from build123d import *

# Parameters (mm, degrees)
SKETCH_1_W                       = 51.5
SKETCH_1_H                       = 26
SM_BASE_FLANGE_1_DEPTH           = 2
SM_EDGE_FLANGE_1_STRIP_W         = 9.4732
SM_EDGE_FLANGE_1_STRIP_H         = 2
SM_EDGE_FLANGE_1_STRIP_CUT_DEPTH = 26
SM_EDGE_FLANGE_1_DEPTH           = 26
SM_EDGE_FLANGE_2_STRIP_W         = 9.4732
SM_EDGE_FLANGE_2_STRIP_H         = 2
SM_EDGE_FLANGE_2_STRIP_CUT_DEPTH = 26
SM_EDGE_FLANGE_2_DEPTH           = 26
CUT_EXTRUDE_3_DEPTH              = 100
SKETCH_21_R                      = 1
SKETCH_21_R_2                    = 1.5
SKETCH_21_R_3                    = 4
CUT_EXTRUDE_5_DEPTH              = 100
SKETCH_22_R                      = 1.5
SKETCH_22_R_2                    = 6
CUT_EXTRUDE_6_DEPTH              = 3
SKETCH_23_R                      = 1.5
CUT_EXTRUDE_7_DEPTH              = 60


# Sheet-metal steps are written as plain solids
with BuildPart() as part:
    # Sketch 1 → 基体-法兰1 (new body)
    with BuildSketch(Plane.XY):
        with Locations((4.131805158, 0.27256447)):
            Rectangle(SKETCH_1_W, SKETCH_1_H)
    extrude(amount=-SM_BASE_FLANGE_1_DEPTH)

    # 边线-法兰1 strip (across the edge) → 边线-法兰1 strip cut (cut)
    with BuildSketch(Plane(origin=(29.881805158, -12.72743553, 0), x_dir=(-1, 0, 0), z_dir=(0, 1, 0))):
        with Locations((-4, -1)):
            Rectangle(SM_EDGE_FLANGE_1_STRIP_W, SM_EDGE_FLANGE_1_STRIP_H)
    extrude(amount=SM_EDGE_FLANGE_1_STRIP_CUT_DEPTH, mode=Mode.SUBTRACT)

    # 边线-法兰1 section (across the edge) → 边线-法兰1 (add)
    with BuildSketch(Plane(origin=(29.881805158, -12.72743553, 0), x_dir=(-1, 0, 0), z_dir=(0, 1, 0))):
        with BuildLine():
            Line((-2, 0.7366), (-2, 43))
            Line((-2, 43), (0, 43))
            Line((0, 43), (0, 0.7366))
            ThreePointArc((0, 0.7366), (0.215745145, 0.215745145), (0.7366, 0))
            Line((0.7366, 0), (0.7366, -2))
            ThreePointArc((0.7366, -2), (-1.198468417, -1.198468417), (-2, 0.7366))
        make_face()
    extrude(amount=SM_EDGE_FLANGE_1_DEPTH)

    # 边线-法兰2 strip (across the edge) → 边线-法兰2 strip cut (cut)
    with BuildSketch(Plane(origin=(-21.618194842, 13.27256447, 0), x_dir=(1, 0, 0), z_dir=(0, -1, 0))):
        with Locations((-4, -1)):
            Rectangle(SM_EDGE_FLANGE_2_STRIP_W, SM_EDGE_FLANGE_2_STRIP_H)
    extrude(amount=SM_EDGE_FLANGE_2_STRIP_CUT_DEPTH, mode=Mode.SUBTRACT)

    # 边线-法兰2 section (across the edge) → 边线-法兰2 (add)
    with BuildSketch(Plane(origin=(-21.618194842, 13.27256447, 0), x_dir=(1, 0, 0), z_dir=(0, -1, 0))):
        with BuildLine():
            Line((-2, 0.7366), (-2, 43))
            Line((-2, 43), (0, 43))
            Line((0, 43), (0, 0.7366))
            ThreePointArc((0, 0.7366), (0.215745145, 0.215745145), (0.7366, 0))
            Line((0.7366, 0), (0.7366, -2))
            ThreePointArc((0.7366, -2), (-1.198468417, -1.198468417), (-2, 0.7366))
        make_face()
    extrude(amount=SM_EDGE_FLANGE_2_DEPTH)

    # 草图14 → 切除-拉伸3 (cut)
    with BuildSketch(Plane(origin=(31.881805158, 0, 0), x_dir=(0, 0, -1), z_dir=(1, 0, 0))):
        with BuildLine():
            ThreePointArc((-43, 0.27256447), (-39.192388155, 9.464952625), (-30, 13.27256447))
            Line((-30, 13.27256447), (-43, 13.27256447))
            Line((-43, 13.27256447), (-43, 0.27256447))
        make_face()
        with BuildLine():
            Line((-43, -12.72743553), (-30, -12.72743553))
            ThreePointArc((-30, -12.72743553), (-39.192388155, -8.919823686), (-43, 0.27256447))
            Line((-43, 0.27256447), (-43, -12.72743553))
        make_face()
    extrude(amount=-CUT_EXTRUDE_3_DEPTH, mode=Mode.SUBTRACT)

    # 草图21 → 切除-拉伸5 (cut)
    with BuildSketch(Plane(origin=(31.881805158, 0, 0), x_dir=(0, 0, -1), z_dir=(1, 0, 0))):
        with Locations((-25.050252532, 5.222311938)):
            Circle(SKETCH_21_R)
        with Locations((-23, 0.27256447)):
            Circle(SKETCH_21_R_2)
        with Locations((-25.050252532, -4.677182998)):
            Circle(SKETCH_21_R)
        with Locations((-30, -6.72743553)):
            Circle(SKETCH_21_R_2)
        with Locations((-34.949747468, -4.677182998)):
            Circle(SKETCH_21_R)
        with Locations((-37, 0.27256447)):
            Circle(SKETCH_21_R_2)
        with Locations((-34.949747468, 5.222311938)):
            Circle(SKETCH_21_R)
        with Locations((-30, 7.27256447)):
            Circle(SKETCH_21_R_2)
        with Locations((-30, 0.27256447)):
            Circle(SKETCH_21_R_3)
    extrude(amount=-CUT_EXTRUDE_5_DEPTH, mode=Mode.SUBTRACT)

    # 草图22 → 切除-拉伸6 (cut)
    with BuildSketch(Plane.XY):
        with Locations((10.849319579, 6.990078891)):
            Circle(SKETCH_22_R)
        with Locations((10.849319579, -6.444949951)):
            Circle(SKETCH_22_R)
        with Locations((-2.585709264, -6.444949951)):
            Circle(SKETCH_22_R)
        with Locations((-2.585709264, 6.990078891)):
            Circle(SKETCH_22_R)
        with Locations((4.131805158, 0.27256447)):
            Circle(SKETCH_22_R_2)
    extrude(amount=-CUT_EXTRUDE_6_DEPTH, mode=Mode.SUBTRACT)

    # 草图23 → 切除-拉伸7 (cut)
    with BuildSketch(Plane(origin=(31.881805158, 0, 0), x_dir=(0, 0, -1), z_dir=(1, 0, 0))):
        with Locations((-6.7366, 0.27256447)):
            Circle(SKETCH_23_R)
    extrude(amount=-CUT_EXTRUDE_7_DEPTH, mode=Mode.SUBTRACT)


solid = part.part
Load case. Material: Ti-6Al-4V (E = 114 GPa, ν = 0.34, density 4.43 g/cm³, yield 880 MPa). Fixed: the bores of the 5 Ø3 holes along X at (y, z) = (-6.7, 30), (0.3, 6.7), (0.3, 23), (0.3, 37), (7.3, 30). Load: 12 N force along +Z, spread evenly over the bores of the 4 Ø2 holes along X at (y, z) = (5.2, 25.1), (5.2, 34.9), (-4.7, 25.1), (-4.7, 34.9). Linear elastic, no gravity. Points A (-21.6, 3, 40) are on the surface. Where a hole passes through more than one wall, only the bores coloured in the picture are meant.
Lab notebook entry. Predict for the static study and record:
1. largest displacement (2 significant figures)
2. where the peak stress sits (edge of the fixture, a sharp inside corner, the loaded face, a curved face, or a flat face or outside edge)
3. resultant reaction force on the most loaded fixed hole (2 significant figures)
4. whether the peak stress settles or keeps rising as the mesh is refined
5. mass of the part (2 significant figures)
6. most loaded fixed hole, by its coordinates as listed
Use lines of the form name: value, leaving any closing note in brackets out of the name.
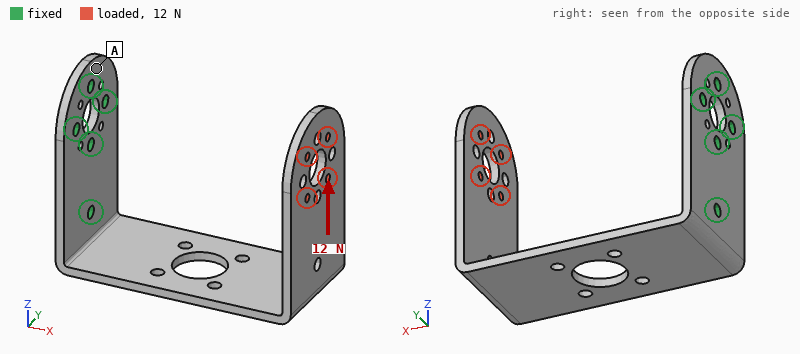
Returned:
largest displacement: 0.75 mm
where the peak stress sits: edge of the fixture
resultant reaction force on the most loaded fixed hole: 20 N
whether the peak stress settles or keeps rising as the mesh is refined: keeps rising
mass of the part: 28 g
most loaded fixed hole, by its coordinates as listed: (0.3, 6.7)
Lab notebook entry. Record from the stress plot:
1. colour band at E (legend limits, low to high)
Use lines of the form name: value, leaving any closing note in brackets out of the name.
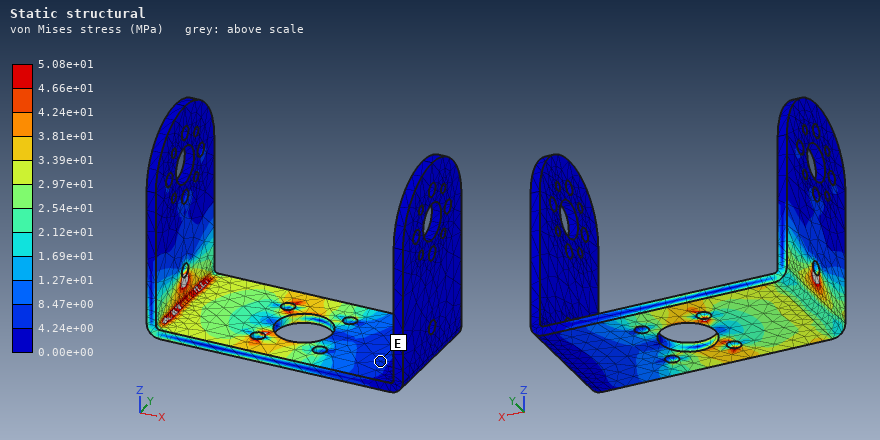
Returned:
colour band at E: 4.24e+00 to 8.47e+00 MPa
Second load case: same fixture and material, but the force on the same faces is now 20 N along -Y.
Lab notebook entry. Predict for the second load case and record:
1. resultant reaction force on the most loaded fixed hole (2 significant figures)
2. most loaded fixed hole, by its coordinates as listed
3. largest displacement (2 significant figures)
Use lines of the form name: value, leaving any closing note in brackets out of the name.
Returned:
resultant reaction force on the most loaded fixed hole: 14 N
most loaded fixed hole, by its coordinates as listed: (0.3, 23)
largest displacement: 0.76 mm
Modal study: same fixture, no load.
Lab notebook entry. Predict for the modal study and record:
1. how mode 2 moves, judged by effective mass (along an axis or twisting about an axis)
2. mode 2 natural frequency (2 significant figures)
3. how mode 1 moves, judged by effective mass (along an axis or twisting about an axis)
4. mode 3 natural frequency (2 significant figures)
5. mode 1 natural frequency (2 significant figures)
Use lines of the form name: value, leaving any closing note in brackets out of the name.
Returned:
how mode 2 moves, judged by effective mass: along Y
mode 2 natural frequency: 370 Hz
how mode 1 moves, judged by effective mass: along Z
mode 3 natural frequency: 690 Hz
mode 1 natural frequency: 210 Hz
